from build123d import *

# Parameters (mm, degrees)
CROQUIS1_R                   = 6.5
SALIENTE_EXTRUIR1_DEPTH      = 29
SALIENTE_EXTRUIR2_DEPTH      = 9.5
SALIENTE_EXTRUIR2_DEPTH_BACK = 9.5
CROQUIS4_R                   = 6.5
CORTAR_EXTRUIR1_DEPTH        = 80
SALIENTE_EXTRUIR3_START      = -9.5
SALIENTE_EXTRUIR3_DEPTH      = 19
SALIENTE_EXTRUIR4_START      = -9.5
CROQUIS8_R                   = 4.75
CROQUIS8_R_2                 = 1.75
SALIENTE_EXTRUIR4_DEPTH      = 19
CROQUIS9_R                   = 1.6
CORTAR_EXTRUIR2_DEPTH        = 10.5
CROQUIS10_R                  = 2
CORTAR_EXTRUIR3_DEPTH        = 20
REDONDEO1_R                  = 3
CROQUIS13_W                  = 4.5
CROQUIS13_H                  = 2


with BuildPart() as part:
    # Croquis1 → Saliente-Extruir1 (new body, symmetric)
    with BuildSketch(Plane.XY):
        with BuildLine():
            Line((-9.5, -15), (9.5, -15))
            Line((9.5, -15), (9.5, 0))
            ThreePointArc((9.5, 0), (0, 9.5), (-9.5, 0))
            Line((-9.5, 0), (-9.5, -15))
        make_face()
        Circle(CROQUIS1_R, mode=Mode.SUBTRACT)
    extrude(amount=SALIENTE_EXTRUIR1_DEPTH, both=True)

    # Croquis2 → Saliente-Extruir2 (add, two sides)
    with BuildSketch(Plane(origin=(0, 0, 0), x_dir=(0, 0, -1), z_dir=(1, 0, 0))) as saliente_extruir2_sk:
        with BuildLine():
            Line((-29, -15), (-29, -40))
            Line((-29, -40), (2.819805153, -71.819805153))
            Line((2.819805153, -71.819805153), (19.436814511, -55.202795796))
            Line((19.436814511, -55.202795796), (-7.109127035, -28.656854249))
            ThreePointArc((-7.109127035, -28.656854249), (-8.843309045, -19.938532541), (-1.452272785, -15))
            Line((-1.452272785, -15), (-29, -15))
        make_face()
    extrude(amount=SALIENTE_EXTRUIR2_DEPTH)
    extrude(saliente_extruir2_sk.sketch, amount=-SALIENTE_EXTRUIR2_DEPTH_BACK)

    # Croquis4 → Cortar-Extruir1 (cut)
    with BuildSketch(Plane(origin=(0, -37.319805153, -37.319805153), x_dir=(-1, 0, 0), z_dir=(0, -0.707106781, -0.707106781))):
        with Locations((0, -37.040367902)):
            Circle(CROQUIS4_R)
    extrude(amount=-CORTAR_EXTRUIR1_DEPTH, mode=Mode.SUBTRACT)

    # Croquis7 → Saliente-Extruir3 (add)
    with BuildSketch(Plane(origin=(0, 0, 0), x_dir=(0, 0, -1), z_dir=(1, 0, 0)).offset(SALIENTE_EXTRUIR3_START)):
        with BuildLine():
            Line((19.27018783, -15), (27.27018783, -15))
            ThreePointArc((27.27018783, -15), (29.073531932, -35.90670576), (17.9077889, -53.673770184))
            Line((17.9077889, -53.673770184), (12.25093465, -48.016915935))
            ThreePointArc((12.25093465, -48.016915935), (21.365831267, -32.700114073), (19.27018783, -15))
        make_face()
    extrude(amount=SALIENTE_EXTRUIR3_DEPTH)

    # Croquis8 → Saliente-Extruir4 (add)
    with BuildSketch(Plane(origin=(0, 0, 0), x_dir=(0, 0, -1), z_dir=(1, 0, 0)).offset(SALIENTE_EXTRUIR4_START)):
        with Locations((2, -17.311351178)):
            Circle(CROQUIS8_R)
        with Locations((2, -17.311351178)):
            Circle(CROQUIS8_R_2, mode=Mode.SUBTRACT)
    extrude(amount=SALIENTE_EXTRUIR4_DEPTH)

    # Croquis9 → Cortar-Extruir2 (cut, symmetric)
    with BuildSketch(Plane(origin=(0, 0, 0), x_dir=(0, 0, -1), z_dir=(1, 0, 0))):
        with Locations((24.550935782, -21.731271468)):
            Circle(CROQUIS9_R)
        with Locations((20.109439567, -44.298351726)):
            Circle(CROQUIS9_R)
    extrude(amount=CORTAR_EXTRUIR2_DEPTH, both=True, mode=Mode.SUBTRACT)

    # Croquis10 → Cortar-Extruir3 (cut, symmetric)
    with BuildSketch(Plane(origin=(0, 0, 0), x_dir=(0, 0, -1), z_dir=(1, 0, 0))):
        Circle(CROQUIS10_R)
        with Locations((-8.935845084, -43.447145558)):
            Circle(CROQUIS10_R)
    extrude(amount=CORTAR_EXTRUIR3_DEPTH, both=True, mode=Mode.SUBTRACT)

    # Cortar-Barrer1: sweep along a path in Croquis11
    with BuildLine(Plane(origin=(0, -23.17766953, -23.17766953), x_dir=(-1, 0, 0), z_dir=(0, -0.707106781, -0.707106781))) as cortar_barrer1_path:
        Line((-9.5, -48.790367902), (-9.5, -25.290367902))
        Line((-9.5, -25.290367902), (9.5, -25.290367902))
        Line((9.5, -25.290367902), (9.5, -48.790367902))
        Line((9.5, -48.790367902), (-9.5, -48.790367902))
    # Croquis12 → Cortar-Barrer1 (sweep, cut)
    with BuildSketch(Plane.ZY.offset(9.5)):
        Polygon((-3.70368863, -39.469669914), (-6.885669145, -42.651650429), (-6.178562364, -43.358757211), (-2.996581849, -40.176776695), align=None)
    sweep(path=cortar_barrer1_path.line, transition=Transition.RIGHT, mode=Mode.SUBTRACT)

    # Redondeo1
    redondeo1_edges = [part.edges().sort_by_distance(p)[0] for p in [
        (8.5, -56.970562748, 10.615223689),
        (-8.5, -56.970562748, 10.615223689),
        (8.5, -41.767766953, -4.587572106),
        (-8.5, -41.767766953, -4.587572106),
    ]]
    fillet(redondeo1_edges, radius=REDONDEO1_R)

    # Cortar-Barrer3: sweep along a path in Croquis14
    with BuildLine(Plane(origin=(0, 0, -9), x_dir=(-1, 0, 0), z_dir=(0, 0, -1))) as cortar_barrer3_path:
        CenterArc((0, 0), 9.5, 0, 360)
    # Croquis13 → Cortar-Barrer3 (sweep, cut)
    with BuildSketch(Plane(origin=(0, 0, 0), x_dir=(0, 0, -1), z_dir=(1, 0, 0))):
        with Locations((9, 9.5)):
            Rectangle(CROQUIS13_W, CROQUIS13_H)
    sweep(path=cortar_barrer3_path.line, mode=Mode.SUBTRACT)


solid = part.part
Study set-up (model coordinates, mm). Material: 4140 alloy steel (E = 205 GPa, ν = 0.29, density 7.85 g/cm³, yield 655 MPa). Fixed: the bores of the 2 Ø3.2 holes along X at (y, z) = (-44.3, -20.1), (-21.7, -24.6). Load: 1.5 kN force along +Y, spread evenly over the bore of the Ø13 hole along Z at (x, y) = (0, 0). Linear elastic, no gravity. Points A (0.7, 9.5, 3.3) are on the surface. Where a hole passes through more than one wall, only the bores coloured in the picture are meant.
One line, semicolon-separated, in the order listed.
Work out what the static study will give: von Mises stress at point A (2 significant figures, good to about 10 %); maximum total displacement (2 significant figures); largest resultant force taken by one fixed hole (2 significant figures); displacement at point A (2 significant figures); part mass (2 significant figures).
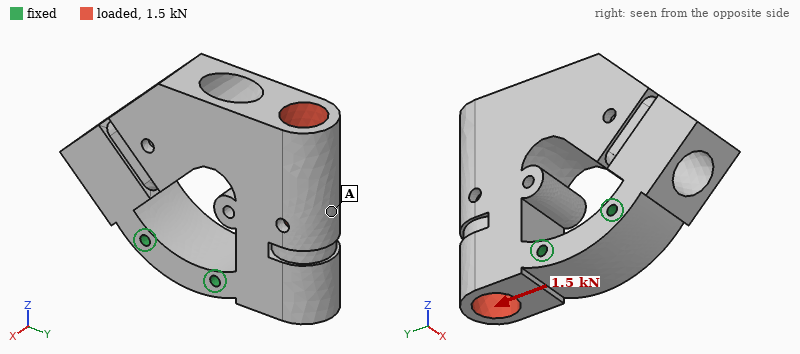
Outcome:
6.1 MPa; 15 µm; 1.2 kN; 12 µm; 330 g
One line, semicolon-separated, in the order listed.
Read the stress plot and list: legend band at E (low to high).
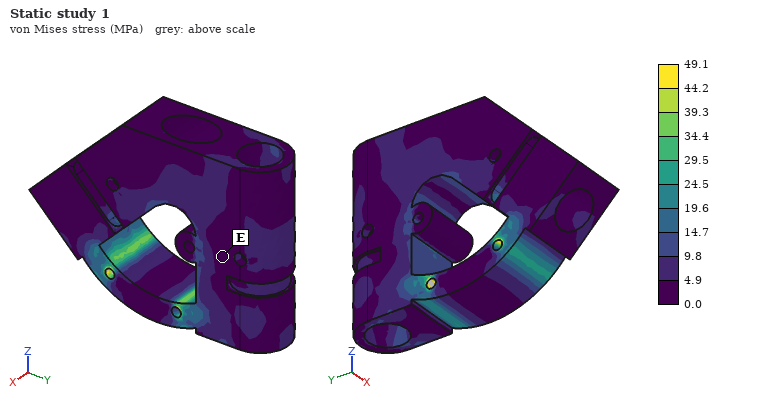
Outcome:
0.0 to 4.9 MPa
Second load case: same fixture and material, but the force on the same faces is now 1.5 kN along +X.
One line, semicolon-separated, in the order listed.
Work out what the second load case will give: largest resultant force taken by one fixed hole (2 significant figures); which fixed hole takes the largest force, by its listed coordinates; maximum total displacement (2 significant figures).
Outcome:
1.4 kN; (-21.7, -24.6); 50 µm
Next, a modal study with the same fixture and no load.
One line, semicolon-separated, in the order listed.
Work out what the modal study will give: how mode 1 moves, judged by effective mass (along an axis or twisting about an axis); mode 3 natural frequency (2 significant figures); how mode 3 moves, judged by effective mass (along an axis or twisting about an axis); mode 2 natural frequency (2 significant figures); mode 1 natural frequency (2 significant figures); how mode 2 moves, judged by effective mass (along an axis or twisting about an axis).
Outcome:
along X; 6100 Hz; twisting about Z; 3200 Hz; 2400 Hz; along Y
